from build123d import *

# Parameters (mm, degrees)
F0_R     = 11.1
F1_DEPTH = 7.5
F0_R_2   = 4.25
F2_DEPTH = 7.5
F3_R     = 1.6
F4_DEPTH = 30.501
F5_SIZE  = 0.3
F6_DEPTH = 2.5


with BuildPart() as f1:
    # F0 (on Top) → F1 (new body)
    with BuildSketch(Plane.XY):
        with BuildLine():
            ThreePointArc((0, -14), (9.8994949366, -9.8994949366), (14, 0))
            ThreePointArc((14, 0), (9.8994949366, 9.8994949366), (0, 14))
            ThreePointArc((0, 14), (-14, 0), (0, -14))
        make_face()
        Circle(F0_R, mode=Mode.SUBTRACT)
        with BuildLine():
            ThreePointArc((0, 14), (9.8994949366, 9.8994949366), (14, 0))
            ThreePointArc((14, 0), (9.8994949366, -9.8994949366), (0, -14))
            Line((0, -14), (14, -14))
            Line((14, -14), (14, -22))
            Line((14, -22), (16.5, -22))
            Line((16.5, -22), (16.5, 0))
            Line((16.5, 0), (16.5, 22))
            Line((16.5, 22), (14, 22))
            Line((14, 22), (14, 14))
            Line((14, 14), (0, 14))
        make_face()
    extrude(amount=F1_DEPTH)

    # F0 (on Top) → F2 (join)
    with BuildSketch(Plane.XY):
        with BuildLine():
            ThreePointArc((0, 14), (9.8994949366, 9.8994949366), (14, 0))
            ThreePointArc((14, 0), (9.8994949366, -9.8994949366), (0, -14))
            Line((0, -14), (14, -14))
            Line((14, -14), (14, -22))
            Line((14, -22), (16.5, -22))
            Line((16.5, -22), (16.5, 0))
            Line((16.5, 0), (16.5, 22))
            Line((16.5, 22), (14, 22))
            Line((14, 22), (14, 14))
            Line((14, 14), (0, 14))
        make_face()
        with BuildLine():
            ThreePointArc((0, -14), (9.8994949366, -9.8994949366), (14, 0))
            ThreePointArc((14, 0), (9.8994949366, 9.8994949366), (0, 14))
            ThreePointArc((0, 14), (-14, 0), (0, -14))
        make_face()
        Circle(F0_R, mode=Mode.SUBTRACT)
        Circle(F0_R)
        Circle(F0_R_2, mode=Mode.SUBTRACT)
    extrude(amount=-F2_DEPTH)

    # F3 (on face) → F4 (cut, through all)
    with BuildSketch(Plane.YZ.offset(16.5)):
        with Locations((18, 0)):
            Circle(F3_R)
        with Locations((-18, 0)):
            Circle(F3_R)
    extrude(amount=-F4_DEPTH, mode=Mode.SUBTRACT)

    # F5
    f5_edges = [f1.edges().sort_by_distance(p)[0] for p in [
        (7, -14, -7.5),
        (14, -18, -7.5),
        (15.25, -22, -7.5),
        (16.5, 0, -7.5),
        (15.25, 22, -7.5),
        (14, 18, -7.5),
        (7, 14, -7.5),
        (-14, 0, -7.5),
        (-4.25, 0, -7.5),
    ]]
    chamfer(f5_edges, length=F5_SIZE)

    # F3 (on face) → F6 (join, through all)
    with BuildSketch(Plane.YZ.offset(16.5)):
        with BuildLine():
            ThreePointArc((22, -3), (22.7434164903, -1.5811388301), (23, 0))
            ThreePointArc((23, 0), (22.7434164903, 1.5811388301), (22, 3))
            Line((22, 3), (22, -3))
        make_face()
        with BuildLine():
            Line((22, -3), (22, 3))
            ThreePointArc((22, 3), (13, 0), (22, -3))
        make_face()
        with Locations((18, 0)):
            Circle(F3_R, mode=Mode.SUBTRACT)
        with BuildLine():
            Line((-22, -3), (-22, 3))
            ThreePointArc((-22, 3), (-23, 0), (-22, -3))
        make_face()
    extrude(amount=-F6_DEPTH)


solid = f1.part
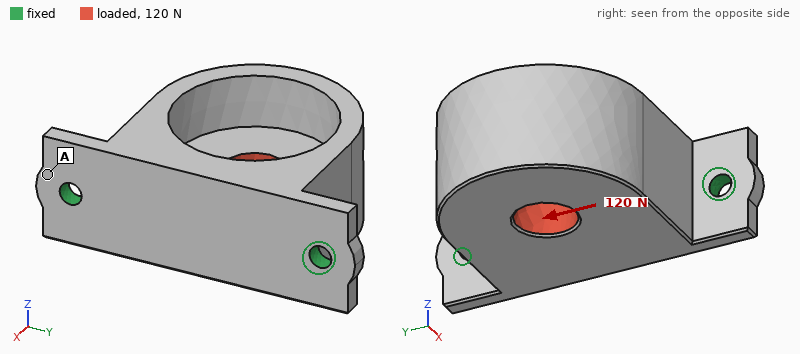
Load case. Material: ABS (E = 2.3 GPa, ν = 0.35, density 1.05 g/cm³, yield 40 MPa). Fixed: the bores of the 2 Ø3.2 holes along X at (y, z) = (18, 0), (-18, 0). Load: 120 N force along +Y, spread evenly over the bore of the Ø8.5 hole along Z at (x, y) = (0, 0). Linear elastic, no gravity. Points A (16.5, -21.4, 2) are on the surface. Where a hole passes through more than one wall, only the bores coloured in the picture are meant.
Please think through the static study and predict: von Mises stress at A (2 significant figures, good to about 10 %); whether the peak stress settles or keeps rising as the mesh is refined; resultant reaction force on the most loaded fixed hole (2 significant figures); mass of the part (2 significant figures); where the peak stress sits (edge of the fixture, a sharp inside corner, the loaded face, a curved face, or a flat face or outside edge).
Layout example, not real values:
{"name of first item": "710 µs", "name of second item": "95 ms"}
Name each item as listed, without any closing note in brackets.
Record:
{"von Mises stress at A": "1.9 MPa", "whether the peak stress settles or keeps rising as the mesh is refined": "keeps rising", "resultant reaction force on the most loaded fixed hole": "85 N", "mass of the part": "9.2 g", "where the peak stress sits": "edge of the fixture"}
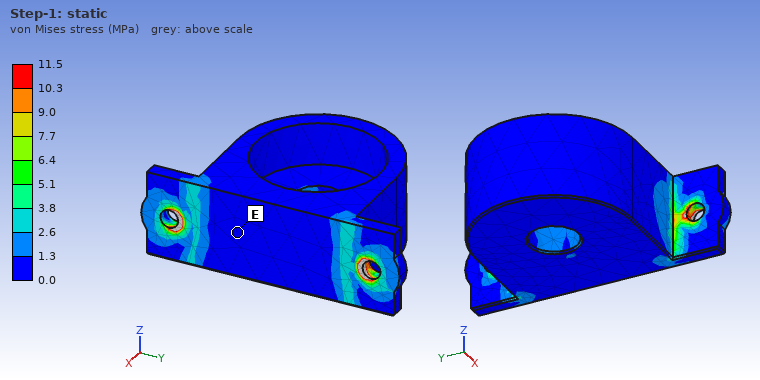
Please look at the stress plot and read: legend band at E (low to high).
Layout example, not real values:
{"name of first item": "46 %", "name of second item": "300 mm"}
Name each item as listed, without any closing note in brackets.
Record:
{"legend band at E": "0.0 to 1.3 MPa"}
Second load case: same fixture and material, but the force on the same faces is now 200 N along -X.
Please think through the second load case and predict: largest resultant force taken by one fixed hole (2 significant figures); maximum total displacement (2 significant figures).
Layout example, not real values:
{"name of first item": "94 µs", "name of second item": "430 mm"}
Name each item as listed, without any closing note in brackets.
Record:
{"largest resultant force taken by one fixed hole": "110 N", "maximum total displacement": "0.58 mm"}
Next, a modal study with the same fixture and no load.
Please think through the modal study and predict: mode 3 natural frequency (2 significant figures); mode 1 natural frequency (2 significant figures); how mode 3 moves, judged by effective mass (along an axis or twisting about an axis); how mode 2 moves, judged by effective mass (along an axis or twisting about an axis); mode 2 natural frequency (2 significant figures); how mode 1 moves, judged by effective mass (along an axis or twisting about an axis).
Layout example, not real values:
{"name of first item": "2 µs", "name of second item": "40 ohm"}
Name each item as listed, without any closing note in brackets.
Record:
{"mode 3 natural frequency": "3200 Hz", "mode 1 natural frequency": "690 Hz", "how mode 3 moves, judged by effective mass": "along X", "how mode 2 moves, judged by effective mass": "along Y", "mode 2 natural frequency": "2700 Hz", "how mode 1 moves, judged by effective mass": "along Z"}
